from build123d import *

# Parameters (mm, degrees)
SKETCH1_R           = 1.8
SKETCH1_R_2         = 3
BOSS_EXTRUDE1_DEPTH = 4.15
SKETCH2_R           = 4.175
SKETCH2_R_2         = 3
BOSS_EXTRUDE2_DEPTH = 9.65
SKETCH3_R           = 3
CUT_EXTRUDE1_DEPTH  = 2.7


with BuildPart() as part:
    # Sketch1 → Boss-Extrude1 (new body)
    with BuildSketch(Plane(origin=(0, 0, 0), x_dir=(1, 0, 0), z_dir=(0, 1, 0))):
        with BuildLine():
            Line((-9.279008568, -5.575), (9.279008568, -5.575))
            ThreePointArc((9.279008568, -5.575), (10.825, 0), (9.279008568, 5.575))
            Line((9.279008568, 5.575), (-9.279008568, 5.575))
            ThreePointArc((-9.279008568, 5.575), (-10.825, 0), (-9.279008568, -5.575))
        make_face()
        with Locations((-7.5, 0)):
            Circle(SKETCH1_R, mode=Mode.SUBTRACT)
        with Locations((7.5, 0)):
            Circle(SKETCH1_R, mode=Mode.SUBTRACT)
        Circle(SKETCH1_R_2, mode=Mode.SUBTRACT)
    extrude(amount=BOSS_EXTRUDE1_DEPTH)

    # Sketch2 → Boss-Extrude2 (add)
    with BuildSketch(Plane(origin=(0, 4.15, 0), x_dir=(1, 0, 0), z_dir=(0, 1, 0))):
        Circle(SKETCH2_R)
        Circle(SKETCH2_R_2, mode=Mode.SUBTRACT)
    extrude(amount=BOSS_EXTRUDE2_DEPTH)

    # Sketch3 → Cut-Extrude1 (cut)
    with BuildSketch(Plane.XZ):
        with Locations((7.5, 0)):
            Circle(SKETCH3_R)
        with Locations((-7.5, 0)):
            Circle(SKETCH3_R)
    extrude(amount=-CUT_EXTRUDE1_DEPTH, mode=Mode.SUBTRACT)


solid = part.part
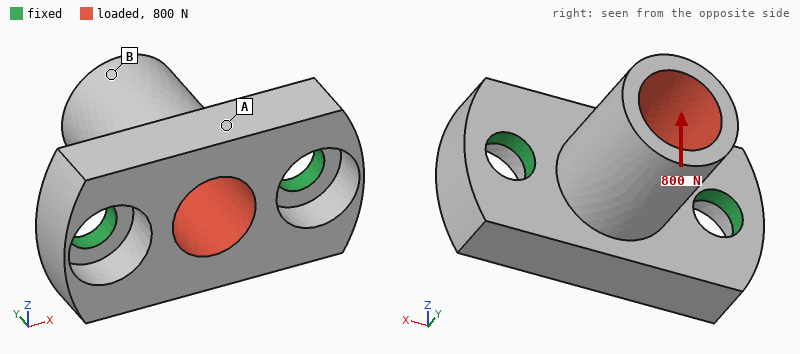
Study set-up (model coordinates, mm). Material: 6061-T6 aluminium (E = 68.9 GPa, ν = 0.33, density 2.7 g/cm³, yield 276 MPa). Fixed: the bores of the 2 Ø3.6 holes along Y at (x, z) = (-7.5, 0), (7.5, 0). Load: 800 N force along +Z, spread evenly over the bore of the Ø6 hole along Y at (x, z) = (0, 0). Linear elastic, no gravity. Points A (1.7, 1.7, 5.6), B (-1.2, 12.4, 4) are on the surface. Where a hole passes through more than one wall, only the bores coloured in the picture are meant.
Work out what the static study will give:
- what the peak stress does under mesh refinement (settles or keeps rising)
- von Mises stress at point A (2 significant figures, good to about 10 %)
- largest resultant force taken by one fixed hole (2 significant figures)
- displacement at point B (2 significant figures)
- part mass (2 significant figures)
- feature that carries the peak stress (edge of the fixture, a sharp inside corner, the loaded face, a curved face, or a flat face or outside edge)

keeps rising
40 MPa
400 N
52 µm
2.5 g
edge of the fixture
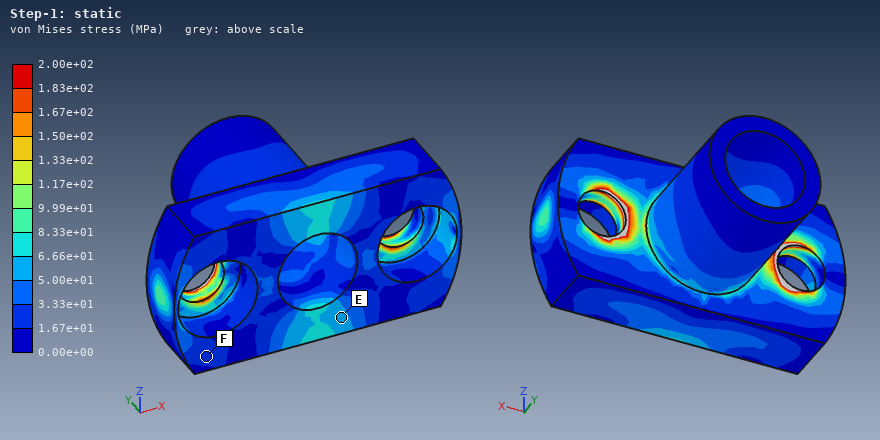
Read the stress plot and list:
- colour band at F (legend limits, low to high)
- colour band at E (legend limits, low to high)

1.67e+01 to 3.33e+01 MPa
5.00e+01 to 6.66e+01 MPa
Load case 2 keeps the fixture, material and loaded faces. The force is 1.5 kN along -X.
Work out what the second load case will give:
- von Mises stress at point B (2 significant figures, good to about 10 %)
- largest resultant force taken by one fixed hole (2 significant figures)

18 MPa
880 N
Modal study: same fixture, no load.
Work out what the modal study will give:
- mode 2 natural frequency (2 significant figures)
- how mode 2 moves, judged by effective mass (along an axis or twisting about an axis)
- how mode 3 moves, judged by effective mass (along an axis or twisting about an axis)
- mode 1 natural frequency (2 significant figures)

33 kHz
along X
along Y
18 kHz
